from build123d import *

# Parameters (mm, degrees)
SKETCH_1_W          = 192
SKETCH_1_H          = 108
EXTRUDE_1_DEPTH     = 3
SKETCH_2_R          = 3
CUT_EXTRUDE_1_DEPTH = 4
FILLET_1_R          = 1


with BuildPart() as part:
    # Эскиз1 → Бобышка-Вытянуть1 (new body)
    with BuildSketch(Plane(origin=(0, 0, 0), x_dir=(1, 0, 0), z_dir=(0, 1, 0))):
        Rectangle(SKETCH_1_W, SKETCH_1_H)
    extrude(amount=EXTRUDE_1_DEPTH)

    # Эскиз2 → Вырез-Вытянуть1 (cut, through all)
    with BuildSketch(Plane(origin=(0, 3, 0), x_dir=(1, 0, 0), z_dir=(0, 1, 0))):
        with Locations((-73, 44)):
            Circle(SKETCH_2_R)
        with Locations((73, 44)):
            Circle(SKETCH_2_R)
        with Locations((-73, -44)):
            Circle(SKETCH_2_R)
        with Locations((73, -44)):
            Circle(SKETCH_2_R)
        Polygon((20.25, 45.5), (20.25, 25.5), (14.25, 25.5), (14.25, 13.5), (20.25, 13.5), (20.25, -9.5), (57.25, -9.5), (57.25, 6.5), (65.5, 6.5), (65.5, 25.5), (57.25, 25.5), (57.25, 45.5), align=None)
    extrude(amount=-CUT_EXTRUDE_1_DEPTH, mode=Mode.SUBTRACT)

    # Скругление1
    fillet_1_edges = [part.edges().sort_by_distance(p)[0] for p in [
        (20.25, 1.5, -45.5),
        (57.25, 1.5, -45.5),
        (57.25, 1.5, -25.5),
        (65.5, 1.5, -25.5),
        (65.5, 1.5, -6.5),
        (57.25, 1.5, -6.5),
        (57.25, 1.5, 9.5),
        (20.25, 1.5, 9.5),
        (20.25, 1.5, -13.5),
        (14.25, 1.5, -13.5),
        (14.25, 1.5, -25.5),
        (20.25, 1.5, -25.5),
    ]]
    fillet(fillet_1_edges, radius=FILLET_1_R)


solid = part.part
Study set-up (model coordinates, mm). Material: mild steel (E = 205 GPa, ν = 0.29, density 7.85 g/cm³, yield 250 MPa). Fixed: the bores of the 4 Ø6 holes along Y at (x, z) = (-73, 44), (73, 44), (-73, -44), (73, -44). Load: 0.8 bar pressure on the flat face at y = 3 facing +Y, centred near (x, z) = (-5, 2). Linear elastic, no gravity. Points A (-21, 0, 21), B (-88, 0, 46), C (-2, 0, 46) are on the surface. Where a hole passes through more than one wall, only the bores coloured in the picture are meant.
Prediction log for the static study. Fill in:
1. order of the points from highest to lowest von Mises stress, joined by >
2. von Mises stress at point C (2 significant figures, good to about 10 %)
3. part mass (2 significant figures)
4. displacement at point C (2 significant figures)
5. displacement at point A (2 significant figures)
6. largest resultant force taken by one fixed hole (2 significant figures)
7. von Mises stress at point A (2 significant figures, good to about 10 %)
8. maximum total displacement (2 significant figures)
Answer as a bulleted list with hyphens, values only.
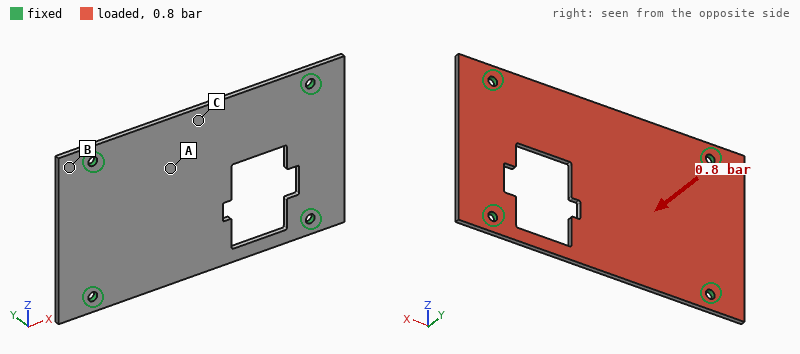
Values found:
- C > A > B
- 54 MPa
- 430 g
- 0.24 mm
- 0.23 mm
- 400 N
- 33 MPa
- 0.32 mm
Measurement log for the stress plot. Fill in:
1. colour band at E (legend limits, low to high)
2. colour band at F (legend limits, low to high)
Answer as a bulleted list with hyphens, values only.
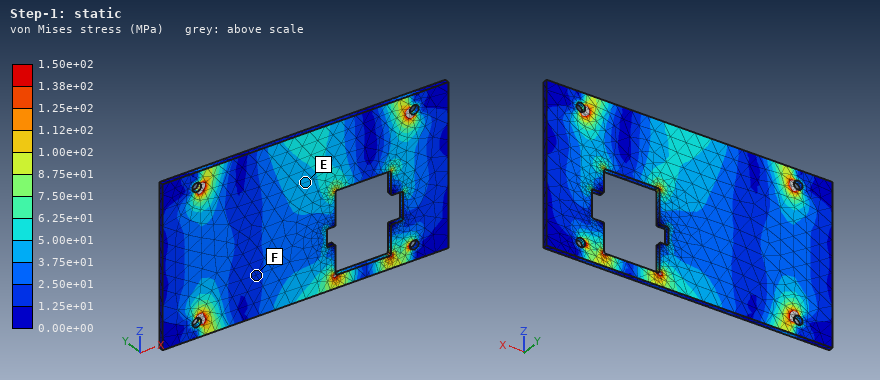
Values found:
- 3.75e+01 to 5.00e+01 MPa
- 1.25e+01 to 2.50e+01 MPa
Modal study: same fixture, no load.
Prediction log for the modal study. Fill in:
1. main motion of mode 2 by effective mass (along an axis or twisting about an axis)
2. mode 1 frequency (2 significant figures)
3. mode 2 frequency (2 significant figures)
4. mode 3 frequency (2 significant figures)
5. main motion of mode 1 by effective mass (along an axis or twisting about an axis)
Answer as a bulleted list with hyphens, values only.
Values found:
- twisting about X
- 620 Hz
- 940 Hz
- 1700 Hz
- along Y
